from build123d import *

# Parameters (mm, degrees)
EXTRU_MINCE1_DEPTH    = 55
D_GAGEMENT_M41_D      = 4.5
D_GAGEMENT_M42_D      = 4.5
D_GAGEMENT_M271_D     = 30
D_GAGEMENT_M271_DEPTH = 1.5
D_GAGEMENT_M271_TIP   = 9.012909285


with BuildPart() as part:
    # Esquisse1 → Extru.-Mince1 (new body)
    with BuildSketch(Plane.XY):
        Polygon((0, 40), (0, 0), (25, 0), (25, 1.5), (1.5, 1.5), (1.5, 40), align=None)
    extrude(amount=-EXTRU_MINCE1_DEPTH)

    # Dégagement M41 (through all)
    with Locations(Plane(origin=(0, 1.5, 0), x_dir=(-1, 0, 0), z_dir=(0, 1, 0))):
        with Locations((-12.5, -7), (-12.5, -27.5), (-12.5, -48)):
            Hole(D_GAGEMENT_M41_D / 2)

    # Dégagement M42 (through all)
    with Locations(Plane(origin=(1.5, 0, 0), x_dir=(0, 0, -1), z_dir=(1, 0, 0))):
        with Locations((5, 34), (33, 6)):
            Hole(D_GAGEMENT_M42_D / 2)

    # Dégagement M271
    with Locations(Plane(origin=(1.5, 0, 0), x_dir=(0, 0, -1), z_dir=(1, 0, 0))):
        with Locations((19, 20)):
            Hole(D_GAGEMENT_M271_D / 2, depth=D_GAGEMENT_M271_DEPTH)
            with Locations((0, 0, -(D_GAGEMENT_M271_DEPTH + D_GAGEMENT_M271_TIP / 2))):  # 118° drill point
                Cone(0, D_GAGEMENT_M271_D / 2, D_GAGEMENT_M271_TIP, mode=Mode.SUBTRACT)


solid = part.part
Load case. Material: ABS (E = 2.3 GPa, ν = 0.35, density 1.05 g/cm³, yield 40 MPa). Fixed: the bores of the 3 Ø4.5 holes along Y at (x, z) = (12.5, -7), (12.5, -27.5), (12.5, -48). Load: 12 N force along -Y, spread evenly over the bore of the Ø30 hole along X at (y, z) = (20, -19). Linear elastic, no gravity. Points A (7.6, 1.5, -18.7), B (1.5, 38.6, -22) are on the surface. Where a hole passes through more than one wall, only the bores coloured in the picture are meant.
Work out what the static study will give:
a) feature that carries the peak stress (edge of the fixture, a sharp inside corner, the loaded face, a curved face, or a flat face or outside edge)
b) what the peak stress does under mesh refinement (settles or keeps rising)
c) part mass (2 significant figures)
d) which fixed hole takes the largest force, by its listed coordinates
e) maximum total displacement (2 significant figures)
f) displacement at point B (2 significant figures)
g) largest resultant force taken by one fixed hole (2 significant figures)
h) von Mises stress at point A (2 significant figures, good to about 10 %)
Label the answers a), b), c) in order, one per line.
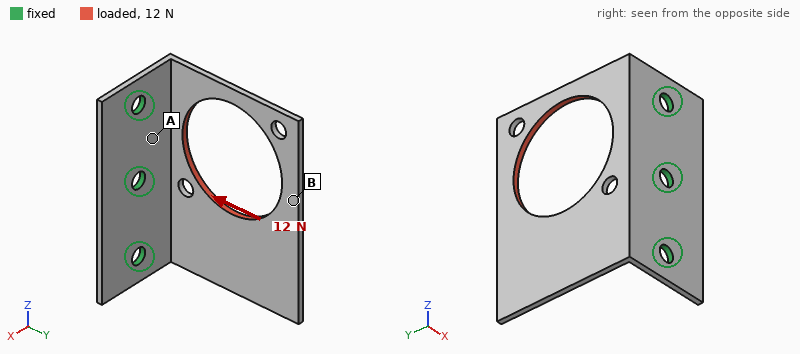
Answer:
a) edge of the fixture
b) keeps rising
c) 4.3 g
d) (12.5, -7)
e) 0.85 mm
f) 0.68 mm
g) 6.3 N
h) 3.0 MPa
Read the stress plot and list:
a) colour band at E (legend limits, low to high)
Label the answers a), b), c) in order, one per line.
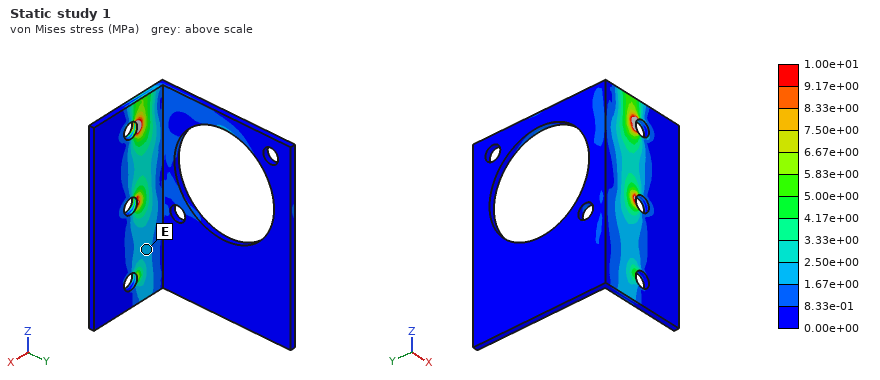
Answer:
a) 1.67e+00 to 2.50e+00 MPa
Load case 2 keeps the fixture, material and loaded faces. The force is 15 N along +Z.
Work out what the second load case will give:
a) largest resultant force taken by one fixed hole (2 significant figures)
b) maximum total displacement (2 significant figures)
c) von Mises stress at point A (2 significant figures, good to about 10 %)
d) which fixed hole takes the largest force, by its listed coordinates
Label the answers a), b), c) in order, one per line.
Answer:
a) 10.0 N
b) 0.69 mm
c) 1.8 MPa
d) (12.5, -7)
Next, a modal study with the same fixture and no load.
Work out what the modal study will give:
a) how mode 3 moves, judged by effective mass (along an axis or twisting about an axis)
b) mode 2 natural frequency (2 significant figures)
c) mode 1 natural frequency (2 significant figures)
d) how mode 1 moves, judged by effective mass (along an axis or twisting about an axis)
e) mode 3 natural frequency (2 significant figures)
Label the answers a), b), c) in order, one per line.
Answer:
a) along Z
b) 330 Hz
c) 160 Hz
d) along X
e) 710 Hz
